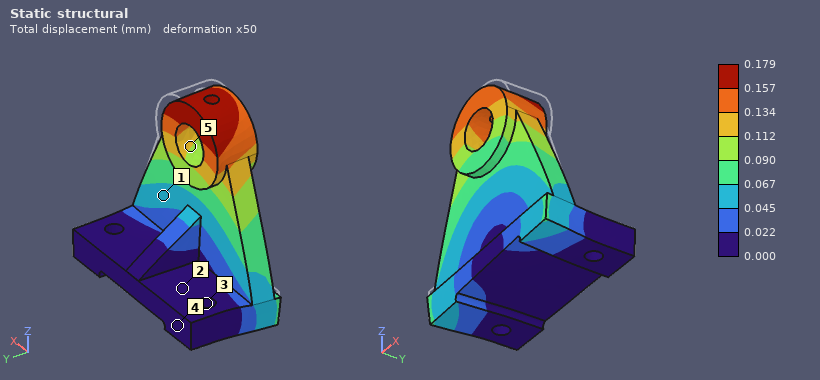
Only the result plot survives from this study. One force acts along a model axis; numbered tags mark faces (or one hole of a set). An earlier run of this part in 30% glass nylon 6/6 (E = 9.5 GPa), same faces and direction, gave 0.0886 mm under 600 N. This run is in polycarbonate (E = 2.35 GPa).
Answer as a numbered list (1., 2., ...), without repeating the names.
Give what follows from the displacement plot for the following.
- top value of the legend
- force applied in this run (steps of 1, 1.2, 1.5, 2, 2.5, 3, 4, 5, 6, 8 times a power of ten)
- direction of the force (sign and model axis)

1. 0.179 mm
2. 300 N
3. -X
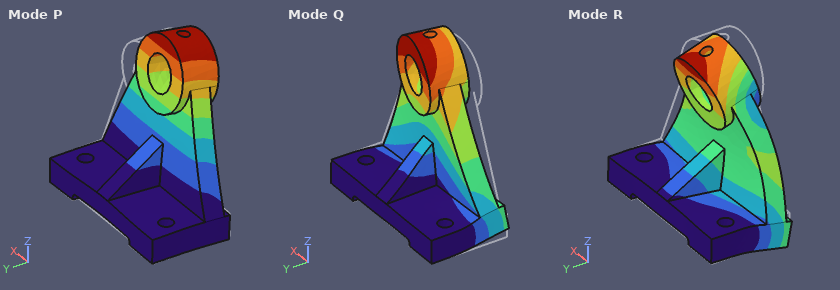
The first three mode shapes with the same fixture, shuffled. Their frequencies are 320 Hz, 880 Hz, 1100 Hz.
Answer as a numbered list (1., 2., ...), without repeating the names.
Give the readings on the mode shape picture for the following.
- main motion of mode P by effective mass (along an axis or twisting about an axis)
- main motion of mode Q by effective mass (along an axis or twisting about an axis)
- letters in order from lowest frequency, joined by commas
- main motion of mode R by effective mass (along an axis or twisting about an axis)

1. along Y
2. along X
3. P, Q, R
4. along Z
